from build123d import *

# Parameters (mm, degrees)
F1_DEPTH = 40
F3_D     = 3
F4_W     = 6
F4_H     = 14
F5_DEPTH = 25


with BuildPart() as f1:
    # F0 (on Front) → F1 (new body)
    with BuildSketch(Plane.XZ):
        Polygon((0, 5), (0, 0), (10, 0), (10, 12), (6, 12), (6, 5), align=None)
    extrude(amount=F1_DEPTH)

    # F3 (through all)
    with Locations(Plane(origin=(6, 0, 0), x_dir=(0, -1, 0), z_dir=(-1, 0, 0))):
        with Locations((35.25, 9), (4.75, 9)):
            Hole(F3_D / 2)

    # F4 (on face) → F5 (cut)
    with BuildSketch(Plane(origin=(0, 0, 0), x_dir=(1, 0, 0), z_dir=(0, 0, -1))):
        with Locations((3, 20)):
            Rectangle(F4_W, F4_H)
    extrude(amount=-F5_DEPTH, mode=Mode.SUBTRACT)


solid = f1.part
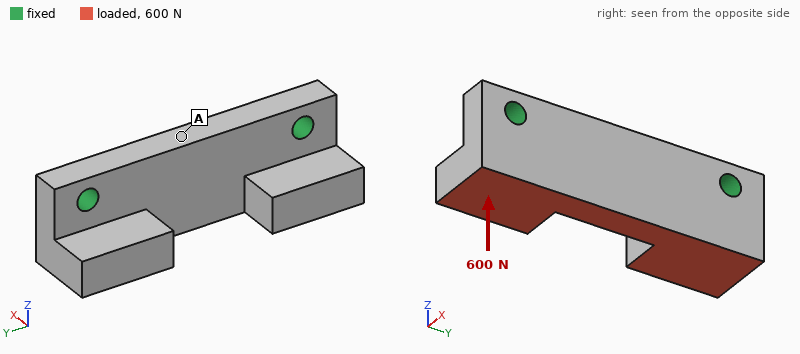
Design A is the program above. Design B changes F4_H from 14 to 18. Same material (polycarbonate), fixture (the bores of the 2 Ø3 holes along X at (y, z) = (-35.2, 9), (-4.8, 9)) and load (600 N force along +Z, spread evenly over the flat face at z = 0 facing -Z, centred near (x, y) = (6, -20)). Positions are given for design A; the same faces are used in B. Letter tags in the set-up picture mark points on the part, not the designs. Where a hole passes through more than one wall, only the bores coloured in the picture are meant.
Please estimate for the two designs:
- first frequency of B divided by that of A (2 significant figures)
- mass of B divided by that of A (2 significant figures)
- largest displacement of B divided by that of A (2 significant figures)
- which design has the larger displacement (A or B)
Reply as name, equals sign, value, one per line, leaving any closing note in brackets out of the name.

first frequency of B divided by that of A = 1.1
mass of B divided by that of A = 0.95
largest displacement of B divided by that of A = 0.91
which design has the larger displacement = A
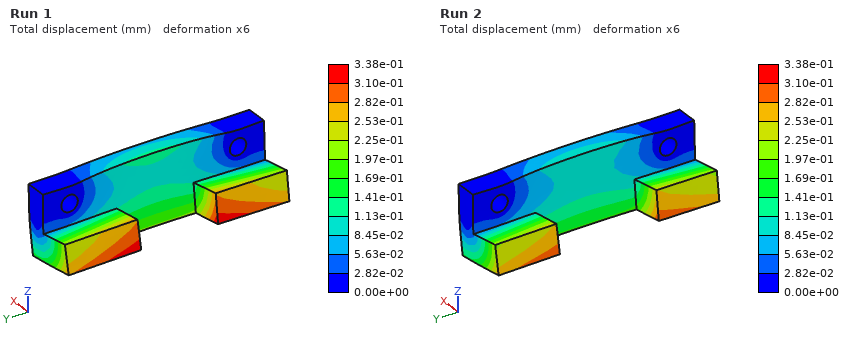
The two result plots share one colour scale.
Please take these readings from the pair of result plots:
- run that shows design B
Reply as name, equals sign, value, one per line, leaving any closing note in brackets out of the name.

run that shows design B = Run 2
